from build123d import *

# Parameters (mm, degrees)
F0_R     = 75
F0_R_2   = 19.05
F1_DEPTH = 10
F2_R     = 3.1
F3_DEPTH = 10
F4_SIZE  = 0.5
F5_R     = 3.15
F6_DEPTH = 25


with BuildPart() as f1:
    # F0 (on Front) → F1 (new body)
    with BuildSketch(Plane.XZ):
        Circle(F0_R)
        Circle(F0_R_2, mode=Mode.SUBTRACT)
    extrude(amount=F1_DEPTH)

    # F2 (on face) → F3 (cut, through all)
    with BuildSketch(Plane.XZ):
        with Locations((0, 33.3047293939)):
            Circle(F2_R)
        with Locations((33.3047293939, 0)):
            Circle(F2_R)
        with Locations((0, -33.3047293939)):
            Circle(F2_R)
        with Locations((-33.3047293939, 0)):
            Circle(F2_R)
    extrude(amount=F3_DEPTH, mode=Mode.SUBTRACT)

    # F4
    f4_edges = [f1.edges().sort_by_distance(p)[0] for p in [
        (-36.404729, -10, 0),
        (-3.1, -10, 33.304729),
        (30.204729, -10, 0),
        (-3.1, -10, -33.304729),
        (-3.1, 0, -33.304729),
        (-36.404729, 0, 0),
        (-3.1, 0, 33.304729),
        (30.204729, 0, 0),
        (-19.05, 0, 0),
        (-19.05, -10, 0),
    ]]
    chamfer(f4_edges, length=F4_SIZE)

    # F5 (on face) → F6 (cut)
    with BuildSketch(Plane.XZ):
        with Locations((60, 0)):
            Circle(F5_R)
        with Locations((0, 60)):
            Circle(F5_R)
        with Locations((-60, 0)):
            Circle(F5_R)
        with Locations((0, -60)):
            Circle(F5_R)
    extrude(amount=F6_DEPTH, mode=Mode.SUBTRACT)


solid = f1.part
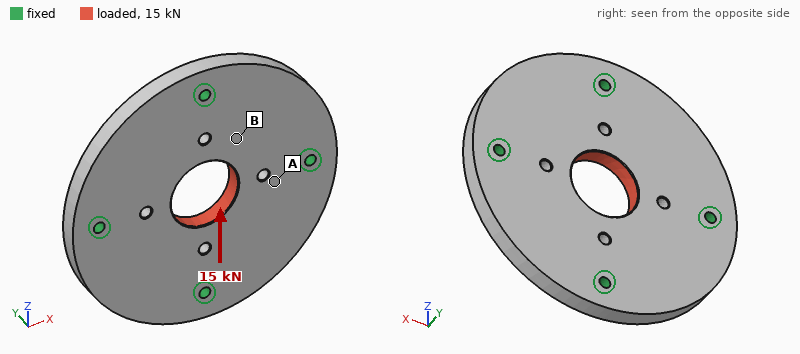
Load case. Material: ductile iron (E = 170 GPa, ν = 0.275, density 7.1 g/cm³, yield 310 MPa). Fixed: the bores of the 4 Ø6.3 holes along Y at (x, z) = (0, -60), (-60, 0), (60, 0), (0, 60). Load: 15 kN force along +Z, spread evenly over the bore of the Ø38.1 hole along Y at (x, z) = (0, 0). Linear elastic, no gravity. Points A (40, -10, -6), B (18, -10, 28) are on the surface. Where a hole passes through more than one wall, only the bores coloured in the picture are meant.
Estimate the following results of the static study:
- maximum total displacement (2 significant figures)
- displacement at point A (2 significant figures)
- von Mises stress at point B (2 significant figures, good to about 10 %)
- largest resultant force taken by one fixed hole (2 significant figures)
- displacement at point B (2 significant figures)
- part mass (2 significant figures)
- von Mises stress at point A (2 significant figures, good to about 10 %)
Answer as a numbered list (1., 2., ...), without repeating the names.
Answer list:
1. 4.6 µm
2. 2.0 µm
3. 11 MPa
4. 4.6 kN
5. 3.2 µm
6. 1.2 kg
7. 3.1 MPa
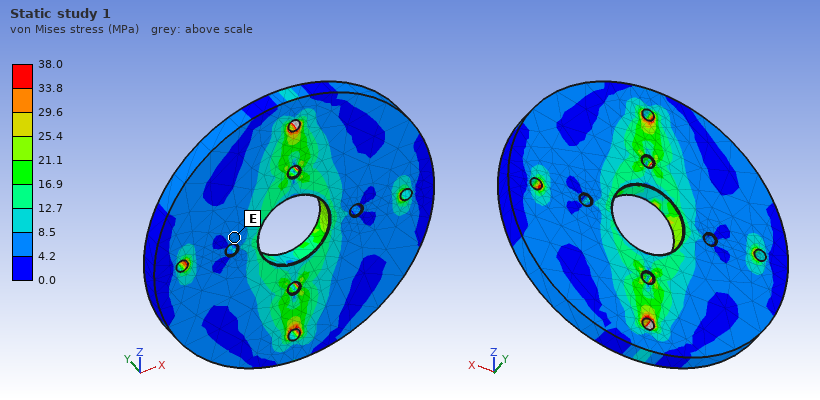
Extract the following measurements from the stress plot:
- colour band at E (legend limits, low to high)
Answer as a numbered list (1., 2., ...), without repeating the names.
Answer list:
1. 4.2 to 8.5 MPa
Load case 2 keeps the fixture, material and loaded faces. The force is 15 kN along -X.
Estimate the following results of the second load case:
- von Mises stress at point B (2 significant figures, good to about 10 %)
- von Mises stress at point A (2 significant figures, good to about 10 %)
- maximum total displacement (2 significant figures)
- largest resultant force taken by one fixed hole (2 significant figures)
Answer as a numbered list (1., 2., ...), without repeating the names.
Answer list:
1. 7.4 MPa
2. 20 MPa
3. 4.6 µm
4. 4.6 kN
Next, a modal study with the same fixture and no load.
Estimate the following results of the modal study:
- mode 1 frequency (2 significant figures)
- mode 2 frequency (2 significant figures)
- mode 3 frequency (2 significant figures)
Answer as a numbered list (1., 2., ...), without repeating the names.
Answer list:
1. 4300 Hz
2. 4800 Hz
3. 4800 Hz
